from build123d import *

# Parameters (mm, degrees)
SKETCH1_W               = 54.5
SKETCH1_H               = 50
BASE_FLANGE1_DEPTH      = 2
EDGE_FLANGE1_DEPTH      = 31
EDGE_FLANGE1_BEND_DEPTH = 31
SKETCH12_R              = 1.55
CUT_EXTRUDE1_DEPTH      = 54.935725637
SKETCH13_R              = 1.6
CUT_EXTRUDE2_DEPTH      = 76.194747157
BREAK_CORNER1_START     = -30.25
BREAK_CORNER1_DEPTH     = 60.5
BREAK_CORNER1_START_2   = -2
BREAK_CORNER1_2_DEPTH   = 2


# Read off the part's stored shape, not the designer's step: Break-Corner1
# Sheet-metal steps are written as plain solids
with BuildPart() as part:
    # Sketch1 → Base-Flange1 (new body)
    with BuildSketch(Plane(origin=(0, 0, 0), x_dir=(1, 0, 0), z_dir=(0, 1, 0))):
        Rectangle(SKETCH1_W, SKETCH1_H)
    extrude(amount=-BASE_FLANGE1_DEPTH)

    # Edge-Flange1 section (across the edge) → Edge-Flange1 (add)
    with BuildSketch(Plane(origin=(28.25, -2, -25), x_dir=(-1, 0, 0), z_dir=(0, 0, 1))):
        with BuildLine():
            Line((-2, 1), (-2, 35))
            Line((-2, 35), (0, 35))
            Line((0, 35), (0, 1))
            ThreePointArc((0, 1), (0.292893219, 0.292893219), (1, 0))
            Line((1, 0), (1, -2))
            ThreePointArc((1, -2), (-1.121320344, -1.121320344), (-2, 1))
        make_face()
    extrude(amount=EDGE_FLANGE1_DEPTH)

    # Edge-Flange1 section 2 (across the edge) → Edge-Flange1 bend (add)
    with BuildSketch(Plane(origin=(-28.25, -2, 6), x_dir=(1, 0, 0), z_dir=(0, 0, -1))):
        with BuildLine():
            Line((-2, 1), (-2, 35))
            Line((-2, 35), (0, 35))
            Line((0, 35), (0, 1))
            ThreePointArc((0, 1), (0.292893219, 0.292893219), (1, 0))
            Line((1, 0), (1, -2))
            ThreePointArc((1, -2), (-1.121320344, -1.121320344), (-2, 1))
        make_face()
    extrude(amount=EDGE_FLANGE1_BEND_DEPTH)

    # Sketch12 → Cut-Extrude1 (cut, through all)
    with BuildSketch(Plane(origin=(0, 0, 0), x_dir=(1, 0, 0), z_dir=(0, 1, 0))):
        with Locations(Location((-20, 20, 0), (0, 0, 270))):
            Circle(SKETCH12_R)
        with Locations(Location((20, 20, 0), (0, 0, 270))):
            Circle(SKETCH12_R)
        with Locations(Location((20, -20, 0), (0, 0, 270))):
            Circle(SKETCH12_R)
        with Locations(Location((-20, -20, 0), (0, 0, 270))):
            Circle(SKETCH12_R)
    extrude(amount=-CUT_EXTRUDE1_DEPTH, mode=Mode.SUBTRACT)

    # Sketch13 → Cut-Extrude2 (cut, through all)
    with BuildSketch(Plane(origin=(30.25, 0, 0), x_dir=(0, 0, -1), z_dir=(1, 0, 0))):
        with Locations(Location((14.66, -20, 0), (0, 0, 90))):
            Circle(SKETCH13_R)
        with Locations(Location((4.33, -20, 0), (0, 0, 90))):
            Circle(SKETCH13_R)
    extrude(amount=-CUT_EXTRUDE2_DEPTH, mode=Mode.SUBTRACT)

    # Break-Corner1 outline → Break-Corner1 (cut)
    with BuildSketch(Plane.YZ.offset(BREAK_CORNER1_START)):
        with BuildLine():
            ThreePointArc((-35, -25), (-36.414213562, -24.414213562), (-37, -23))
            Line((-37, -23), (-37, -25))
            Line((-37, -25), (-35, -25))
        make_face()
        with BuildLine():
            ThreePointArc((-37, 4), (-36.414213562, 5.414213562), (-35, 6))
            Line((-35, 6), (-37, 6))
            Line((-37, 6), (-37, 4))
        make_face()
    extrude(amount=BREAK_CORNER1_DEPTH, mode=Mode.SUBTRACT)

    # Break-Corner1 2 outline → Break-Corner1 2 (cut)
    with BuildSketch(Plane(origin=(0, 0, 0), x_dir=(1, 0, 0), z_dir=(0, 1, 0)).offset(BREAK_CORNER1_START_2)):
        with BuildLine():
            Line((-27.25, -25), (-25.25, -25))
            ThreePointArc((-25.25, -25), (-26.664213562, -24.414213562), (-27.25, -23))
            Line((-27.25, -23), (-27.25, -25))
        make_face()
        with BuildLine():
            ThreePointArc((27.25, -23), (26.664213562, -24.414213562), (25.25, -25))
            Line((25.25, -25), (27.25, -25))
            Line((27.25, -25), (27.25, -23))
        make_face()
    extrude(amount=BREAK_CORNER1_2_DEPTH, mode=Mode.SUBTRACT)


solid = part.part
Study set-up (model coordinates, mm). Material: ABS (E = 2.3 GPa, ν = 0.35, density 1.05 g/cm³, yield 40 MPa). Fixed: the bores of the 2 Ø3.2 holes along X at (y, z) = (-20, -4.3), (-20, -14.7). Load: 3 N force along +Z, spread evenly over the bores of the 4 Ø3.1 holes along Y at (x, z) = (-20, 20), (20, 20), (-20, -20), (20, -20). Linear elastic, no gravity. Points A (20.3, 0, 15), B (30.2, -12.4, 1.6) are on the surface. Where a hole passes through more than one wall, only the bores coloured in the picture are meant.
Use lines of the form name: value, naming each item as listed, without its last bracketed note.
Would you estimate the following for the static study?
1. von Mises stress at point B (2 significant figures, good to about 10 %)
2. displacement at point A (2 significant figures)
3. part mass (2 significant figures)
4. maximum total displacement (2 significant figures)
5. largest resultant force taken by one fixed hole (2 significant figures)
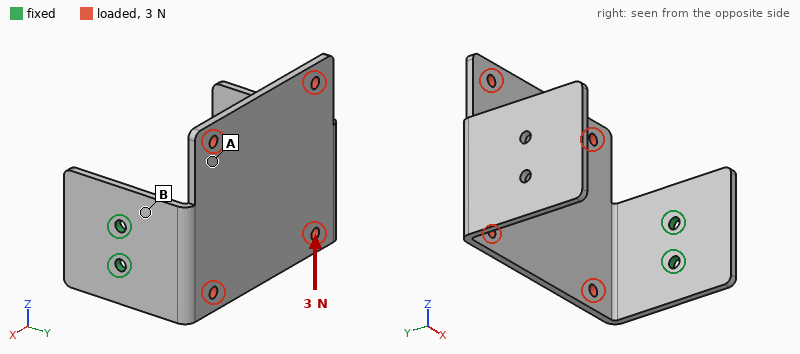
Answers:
von Mises stress at point B: 1.9 MPa
displacement at point A: 0.36 mm
part mass: 10 g
maximum total displacement: 1.00 mm
largest resultant force taken by one fixed hole: 7.1 N
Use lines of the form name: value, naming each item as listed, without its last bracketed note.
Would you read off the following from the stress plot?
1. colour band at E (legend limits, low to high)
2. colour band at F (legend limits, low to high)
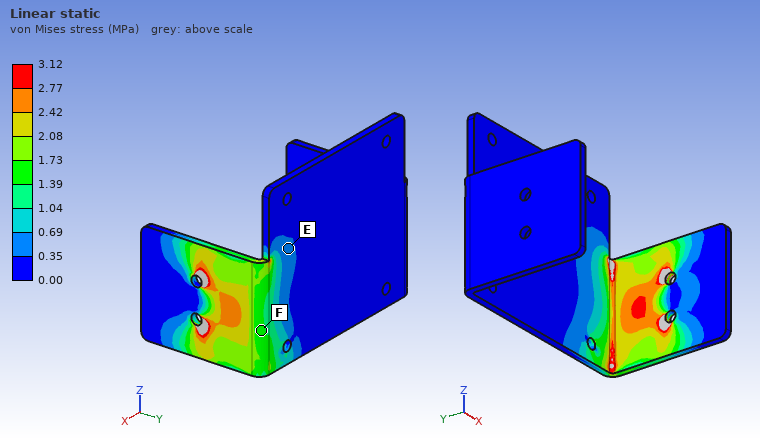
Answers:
colour band at E: 0.35 to 0.69 MPa
colour band at F: 1.39 to 1.73 MPa
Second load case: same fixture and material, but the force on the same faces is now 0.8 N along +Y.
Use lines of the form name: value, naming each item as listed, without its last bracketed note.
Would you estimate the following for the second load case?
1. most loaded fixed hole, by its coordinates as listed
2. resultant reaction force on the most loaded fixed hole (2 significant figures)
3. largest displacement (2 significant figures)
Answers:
most loaded fixed hole, by its coordinates as listed: (-20, -4.3)
resultant reaction force on the most loaded fixed hole: 1.0 N
largest displacement: 0.99 mm
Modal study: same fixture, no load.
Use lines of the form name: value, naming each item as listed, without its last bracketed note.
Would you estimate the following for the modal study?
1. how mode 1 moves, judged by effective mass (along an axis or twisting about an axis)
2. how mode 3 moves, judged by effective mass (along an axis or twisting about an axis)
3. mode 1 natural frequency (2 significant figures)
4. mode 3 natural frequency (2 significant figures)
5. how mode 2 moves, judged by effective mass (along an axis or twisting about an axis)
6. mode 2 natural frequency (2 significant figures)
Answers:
how mode 1 moves, judged by effective mass: along Y
how mode 3 moves, judged by effective mass: along X
mode 1 natural frequency: 51 Hz
mode 3 natural frequency: 190 Hz
how mode 2 moves, judged by effective mass: along Z
mode 2 natural frequency: 90 Hz
